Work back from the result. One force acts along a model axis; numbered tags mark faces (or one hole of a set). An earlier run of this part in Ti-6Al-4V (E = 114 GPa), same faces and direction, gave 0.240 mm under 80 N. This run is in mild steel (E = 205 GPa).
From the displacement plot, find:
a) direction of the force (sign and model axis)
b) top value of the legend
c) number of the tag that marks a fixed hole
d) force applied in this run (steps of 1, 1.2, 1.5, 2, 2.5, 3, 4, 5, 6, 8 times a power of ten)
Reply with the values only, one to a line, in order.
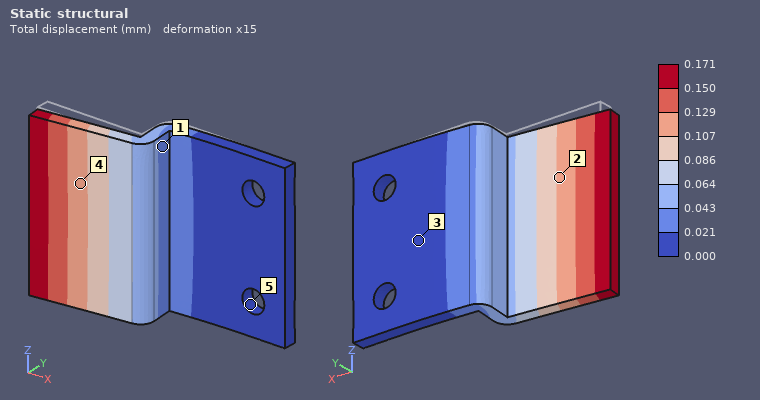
-Y
0.171 mm
5
100 N
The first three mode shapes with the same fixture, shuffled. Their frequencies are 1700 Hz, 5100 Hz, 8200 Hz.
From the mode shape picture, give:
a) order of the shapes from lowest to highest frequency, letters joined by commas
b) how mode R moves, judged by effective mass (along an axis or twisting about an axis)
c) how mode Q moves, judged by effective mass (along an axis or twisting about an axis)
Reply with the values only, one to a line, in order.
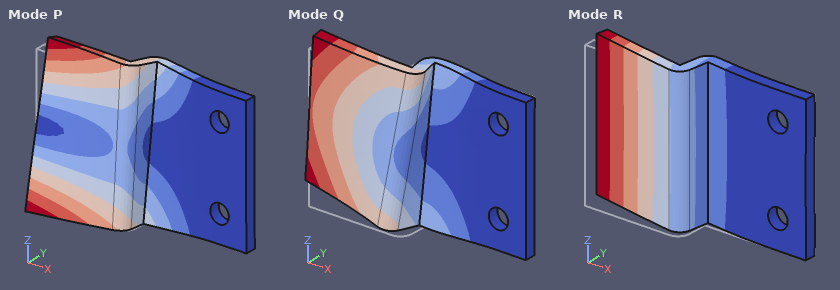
R, P, Q
along Y
along Z
